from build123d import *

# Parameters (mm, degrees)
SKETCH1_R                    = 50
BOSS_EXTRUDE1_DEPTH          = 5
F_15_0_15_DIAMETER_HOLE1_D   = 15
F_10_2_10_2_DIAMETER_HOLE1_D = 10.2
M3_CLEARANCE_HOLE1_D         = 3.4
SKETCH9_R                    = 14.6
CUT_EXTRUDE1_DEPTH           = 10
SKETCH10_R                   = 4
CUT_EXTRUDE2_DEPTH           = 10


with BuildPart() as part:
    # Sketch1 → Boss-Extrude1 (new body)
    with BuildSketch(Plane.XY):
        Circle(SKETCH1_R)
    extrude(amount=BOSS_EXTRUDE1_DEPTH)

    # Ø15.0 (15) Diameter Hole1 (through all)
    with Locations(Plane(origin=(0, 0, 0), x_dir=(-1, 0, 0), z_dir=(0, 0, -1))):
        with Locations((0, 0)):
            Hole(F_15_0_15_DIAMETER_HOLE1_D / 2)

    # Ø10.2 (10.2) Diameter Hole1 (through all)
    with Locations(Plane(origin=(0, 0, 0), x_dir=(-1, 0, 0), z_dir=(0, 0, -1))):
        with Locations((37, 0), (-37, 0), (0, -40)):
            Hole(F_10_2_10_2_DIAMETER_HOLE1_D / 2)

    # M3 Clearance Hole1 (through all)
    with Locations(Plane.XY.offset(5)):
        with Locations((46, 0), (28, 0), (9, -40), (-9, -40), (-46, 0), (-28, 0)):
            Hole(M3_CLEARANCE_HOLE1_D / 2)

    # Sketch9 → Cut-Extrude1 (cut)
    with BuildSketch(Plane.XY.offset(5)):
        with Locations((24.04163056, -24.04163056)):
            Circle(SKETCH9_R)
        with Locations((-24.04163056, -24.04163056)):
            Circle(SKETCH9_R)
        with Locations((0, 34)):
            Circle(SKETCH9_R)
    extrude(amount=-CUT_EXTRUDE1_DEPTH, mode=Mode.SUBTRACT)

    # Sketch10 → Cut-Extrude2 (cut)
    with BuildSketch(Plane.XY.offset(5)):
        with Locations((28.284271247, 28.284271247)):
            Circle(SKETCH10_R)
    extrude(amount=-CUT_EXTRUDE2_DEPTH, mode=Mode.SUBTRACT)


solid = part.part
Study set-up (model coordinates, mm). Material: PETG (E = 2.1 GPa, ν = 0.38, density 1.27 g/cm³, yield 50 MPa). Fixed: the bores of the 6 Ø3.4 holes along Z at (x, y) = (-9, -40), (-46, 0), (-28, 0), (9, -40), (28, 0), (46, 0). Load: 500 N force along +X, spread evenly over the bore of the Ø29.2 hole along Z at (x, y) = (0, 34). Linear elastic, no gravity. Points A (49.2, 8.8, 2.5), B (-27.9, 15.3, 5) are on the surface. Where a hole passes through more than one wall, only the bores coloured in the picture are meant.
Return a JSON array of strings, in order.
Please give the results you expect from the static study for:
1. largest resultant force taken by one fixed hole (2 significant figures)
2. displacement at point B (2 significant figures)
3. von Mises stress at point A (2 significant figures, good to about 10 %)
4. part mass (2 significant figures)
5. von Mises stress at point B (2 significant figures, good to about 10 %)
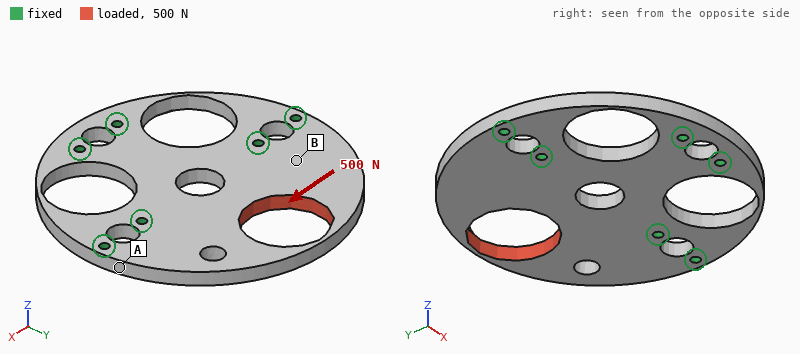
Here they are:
["200 N", "0.036 mm", "2.7 MPa", "34 g", "0.96 MPa"]
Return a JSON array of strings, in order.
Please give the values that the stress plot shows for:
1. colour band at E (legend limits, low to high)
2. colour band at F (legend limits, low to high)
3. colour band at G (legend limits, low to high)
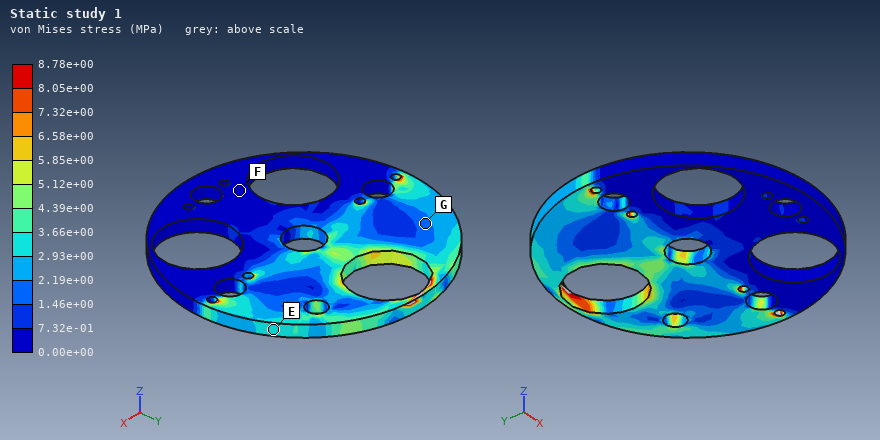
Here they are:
["2.93e+00 to 3.66e+00 MPa", "0.00e+00 to 7.32e-01 MPa", "1.46e+00 to 2.19e+00 MPa"]
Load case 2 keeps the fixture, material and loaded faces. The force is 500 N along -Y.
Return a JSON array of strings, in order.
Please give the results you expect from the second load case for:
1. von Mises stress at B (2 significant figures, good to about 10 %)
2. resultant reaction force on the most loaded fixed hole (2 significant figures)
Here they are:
["1.6 MPa", "170 N"]
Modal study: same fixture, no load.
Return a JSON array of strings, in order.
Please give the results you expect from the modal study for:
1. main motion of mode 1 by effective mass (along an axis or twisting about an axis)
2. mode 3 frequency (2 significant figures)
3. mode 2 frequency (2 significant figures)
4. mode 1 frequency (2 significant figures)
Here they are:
["along Z", "1700 Hz", "930 Hz", "550 Hz"]
